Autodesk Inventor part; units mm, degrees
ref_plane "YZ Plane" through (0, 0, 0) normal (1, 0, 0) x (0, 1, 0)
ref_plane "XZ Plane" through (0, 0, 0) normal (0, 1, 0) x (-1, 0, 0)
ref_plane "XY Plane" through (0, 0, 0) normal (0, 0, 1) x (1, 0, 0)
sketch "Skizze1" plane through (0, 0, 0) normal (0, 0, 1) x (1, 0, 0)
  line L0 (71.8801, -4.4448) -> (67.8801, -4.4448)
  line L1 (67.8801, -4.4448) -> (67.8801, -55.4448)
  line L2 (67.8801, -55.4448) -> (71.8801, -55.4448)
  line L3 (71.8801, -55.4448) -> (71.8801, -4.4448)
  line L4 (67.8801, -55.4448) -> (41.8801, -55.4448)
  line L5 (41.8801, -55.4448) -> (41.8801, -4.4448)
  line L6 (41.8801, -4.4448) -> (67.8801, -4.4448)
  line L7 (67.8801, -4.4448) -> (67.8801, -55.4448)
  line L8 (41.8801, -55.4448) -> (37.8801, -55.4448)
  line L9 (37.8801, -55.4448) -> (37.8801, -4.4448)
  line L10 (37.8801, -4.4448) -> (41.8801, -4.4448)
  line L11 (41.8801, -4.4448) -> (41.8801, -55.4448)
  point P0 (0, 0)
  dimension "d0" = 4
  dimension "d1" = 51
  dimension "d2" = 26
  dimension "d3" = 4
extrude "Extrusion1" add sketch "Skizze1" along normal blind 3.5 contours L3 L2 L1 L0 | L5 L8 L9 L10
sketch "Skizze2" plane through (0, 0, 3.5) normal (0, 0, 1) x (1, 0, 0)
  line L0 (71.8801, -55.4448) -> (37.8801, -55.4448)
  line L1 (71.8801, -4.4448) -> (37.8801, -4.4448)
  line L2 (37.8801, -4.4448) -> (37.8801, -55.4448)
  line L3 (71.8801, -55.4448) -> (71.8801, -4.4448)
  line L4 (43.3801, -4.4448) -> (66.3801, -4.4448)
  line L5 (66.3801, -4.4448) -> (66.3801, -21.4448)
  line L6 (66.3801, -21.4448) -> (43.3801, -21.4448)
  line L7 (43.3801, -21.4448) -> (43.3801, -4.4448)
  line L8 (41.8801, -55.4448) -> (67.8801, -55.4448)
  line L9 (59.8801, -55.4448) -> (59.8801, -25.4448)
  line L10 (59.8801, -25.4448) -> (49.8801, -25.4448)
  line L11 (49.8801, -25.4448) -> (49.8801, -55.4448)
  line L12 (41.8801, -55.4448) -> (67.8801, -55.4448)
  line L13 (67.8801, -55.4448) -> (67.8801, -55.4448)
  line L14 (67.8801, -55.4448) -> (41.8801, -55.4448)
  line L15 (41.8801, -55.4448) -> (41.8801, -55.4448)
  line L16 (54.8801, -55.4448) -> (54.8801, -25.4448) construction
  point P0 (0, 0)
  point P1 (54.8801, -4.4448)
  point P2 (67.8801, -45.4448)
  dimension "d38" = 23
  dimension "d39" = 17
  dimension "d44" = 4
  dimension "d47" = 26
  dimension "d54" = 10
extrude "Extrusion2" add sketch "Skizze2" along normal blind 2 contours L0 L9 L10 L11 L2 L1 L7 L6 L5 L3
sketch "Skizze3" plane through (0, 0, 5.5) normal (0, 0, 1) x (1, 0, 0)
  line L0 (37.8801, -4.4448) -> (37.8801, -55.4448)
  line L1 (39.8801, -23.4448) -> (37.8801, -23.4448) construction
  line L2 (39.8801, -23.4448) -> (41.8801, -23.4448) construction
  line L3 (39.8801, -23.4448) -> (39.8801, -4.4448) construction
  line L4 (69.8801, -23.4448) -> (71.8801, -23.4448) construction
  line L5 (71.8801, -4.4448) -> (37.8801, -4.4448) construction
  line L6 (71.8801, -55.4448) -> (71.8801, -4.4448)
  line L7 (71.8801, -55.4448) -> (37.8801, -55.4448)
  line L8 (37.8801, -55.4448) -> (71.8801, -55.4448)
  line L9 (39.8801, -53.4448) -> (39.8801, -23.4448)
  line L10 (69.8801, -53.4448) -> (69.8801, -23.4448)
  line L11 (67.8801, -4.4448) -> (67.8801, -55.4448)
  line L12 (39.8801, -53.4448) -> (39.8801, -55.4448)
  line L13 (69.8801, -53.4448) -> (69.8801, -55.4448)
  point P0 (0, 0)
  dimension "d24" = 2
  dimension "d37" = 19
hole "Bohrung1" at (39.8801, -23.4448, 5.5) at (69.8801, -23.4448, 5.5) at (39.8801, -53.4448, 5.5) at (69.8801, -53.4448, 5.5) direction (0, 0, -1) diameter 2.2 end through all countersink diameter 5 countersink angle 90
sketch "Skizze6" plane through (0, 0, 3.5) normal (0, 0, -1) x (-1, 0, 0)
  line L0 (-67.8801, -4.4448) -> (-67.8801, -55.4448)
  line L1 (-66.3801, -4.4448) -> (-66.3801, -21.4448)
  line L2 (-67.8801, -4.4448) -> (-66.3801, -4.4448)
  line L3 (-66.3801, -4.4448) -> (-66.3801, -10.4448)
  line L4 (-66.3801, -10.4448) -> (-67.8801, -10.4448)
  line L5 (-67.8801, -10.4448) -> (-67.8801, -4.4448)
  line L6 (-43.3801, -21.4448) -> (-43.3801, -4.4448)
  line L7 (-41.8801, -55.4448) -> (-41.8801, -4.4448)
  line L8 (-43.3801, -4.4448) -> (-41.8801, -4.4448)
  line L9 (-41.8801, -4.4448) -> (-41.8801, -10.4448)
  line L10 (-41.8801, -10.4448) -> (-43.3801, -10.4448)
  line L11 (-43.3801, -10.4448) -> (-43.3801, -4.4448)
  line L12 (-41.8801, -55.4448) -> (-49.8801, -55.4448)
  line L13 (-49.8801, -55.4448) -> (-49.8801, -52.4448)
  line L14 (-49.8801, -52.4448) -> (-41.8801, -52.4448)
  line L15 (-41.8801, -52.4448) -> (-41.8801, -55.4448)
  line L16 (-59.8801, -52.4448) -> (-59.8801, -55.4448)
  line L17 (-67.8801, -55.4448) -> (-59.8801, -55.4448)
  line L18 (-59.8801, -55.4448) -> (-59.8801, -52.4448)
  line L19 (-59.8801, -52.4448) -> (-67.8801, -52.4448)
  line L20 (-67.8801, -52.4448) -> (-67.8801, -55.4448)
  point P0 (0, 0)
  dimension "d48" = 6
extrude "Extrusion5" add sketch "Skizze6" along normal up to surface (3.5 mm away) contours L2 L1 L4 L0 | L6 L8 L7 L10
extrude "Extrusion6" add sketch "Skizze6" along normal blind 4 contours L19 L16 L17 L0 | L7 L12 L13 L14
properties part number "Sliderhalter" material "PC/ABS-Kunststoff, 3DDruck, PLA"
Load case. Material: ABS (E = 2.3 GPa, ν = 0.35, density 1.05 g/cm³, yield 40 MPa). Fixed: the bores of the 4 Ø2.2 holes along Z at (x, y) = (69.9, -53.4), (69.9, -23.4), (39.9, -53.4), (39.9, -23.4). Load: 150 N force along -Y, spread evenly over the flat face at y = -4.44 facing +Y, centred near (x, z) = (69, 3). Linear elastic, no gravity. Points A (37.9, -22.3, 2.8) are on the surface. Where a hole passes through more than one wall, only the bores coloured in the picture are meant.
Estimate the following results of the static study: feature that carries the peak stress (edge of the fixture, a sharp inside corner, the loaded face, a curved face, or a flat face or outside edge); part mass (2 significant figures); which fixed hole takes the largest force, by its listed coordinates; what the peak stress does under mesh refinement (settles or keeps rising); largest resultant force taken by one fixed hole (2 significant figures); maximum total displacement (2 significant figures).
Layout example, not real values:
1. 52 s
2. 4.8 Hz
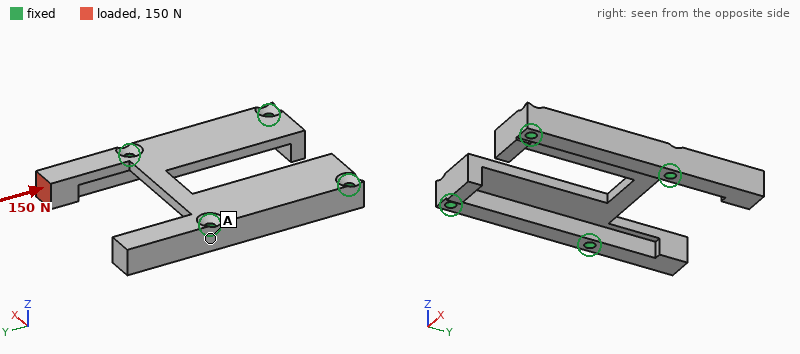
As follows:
1. edge of the fixture
2. 3.8 g
3. (69.9, -23.4)
4. keeps rising
5. 140 N
6. 0.15 mm
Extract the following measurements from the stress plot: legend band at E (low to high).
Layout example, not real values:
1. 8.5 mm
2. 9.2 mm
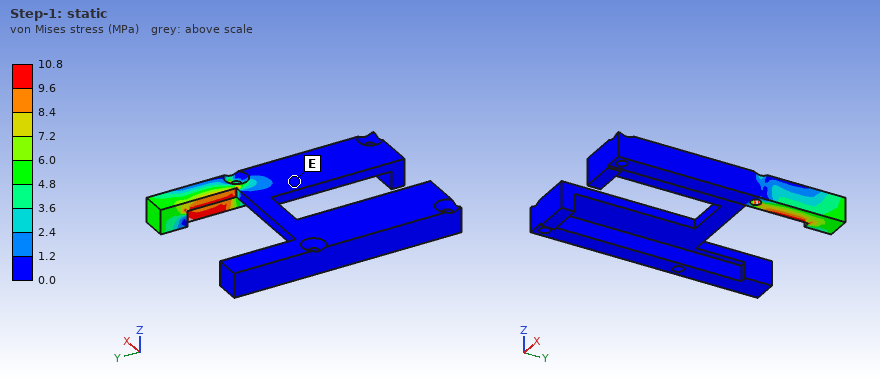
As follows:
1. 0.0 to 1.2 MPa
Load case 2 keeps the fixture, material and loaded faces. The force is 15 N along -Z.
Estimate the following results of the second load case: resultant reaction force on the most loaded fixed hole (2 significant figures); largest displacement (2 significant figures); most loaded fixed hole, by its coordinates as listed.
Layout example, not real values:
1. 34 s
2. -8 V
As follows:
1. 17 N
2. 0.31 mm
3. (69.9, -23.4)
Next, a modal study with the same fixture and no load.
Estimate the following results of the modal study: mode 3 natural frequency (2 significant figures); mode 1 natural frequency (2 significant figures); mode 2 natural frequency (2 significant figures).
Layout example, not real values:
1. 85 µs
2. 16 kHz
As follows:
1. 3200 Hz
2. 2500 Hz
3. 2500 Hz
